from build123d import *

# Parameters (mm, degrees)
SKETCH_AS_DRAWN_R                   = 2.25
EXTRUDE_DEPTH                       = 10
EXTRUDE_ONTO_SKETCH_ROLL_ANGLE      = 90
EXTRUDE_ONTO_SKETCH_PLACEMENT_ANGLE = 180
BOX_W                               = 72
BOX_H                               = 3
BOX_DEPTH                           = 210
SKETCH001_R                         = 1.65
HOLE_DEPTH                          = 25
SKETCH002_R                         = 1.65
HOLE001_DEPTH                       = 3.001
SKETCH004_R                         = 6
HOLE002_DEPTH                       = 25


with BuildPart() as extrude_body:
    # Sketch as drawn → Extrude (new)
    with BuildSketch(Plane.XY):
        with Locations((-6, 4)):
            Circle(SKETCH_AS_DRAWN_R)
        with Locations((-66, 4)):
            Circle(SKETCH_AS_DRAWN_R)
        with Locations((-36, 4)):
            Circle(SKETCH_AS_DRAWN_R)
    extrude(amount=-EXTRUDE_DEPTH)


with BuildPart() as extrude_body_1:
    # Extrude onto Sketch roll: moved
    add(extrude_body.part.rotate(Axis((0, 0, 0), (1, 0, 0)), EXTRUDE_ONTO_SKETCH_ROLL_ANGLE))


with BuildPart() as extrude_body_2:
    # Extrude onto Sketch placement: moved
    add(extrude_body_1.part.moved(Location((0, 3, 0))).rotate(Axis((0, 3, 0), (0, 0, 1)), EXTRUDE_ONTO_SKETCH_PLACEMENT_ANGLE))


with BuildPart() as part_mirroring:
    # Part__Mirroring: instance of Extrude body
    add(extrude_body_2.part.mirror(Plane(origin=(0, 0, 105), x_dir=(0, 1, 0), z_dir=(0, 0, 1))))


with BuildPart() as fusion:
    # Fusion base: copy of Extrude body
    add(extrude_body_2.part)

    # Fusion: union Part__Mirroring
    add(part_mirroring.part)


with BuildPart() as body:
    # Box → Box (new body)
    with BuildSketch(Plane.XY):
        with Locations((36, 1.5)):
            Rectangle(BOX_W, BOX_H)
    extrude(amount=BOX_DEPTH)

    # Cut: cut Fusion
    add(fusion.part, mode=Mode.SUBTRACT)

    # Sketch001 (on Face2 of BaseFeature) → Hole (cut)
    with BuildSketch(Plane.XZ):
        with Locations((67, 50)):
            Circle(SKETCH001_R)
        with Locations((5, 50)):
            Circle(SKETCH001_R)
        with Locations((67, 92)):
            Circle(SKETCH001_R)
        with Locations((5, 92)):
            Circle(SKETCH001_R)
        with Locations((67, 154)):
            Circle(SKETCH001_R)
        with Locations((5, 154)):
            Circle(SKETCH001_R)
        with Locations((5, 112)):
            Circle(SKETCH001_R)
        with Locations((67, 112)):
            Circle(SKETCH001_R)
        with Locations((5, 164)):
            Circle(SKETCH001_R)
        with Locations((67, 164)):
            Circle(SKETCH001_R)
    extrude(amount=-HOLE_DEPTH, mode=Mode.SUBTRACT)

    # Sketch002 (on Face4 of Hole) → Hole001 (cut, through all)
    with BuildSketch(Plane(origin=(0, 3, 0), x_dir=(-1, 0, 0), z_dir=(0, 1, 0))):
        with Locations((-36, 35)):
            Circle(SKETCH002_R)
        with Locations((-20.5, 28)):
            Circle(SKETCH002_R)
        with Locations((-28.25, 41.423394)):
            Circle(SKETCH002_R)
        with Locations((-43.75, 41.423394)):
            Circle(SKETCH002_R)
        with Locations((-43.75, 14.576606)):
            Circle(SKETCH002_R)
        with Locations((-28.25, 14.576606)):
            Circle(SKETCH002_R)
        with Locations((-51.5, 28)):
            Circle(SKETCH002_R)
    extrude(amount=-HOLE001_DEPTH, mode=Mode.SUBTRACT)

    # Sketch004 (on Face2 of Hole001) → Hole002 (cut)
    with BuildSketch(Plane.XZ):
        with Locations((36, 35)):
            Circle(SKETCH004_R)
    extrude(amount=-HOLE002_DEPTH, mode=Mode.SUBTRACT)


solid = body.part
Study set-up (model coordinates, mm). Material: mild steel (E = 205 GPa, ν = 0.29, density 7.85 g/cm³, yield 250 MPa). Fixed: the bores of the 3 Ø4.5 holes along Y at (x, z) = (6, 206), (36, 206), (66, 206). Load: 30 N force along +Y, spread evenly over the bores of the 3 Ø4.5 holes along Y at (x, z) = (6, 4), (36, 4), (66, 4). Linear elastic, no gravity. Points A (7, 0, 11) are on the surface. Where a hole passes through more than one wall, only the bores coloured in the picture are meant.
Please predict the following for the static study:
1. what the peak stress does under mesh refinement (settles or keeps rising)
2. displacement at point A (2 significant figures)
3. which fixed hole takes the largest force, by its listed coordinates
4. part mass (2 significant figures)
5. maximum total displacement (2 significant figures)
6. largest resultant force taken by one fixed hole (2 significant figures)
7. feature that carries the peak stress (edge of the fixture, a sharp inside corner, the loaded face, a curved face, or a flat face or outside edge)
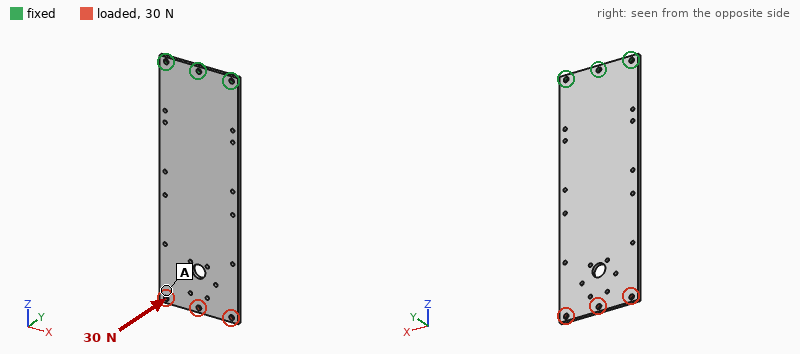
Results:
keeps rising
2.4 mm
(36, 206)
350 g
2.6 mm
57 N
edge of the fixture
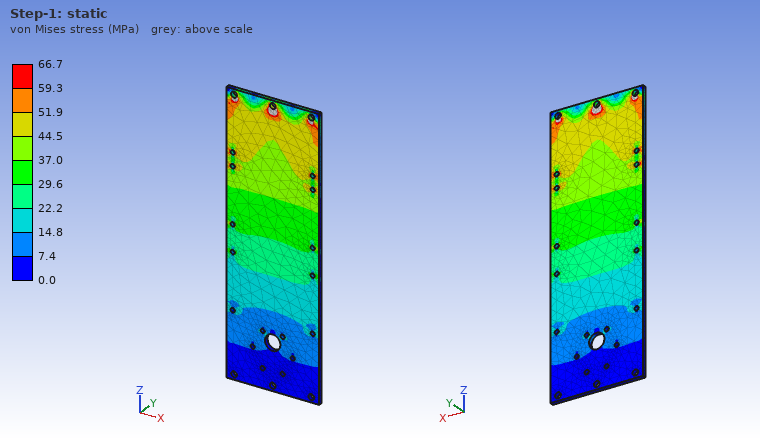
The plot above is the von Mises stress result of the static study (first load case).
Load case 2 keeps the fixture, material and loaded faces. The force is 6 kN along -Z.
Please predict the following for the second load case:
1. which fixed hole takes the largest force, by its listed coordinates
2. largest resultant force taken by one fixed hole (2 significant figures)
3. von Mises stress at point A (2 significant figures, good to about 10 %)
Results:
(36, 206)
2.3 kN
47 MPa
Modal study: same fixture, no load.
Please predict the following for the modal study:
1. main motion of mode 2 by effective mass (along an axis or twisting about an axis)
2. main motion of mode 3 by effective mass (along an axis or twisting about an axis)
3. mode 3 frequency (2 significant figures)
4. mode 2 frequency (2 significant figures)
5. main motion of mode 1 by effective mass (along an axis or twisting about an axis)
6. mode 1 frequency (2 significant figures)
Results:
twisting about Z
along Y
370 Hz
350 Hz
along Y
59 Hz
